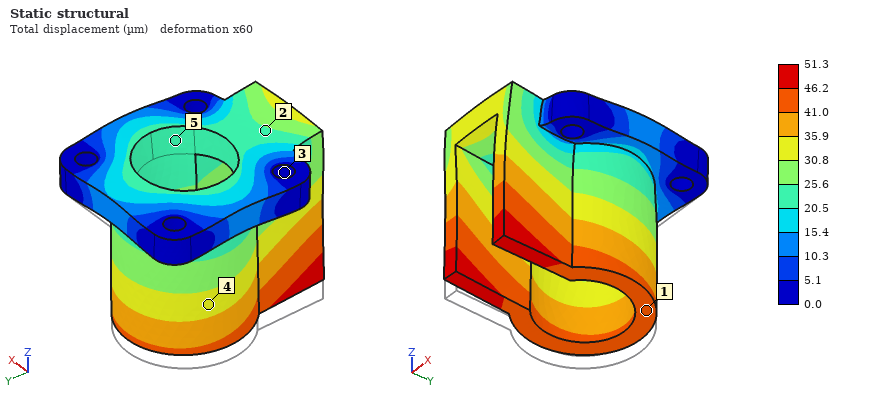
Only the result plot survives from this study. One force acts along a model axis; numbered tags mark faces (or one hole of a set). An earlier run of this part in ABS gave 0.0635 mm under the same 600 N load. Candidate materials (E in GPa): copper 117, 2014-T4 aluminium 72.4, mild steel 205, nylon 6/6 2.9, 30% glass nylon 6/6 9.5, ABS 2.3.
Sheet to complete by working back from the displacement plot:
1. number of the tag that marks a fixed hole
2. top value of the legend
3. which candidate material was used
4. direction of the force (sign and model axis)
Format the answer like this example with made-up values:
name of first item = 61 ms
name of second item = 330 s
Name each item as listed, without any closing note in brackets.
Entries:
number of the tag that marks a fixed hole = 3
top value of the legend = 51.3 µm
which candidate material was used = nylon 6/6
direction of the force = +Z
